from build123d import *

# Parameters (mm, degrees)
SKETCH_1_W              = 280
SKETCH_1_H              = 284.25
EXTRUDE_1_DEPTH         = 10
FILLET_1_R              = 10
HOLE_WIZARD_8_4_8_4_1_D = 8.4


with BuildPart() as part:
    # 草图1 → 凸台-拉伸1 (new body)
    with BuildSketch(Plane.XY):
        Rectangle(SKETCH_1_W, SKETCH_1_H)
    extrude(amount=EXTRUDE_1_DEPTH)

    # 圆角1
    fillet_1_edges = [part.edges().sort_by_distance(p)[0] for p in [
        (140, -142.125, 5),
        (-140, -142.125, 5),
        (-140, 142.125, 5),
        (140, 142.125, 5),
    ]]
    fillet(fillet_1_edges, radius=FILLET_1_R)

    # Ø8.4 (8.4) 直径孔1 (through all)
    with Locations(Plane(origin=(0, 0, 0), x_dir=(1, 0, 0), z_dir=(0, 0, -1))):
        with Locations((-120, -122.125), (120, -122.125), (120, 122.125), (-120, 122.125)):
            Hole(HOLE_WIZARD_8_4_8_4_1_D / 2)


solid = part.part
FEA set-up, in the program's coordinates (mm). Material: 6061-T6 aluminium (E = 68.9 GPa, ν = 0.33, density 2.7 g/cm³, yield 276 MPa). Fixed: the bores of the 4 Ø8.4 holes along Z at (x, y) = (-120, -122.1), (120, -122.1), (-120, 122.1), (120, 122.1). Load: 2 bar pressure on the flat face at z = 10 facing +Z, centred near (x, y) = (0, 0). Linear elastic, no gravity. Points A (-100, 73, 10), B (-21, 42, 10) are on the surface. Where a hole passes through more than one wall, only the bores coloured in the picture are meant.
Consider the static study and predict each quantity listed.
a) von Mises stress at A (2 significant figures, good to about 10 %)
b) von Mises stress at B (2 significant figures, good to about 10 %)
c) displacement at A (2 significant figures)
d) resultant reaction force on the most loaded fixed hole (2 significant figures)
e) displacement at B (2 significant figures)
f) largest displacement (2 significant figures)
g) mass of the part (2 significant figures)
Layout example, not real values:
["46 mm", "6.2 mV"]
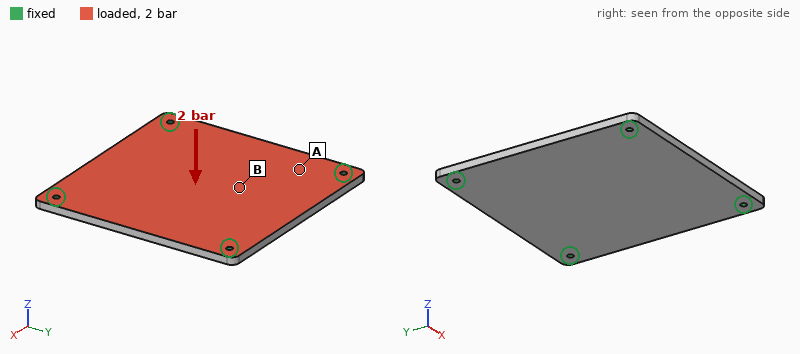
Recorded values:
["15 MPa", "38 MPa", "0.36 mm", "4.0 kN", "0.85 mm", "0.94 mm", "2.1 kg"]
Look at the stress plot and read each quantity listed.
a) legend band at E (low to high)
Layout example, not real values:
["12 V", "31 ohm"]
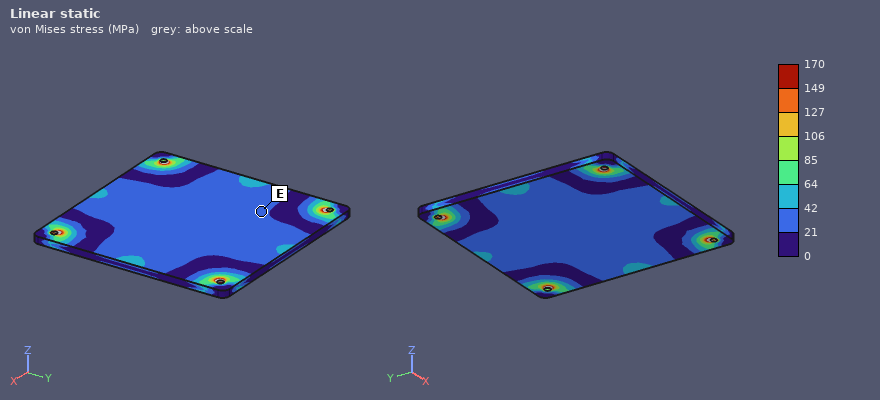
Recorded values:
["21 to 42 MPa"]
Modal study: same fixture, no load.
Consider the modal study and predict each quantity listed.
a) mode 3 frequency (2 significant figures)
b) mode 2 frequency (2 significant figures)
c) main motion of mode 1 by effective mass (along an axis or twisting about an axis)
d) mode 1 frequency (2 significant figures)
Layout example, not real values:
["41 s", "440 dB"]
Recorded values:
["940 Hz", "920 Hz", "along Z", "540 Hz"]
